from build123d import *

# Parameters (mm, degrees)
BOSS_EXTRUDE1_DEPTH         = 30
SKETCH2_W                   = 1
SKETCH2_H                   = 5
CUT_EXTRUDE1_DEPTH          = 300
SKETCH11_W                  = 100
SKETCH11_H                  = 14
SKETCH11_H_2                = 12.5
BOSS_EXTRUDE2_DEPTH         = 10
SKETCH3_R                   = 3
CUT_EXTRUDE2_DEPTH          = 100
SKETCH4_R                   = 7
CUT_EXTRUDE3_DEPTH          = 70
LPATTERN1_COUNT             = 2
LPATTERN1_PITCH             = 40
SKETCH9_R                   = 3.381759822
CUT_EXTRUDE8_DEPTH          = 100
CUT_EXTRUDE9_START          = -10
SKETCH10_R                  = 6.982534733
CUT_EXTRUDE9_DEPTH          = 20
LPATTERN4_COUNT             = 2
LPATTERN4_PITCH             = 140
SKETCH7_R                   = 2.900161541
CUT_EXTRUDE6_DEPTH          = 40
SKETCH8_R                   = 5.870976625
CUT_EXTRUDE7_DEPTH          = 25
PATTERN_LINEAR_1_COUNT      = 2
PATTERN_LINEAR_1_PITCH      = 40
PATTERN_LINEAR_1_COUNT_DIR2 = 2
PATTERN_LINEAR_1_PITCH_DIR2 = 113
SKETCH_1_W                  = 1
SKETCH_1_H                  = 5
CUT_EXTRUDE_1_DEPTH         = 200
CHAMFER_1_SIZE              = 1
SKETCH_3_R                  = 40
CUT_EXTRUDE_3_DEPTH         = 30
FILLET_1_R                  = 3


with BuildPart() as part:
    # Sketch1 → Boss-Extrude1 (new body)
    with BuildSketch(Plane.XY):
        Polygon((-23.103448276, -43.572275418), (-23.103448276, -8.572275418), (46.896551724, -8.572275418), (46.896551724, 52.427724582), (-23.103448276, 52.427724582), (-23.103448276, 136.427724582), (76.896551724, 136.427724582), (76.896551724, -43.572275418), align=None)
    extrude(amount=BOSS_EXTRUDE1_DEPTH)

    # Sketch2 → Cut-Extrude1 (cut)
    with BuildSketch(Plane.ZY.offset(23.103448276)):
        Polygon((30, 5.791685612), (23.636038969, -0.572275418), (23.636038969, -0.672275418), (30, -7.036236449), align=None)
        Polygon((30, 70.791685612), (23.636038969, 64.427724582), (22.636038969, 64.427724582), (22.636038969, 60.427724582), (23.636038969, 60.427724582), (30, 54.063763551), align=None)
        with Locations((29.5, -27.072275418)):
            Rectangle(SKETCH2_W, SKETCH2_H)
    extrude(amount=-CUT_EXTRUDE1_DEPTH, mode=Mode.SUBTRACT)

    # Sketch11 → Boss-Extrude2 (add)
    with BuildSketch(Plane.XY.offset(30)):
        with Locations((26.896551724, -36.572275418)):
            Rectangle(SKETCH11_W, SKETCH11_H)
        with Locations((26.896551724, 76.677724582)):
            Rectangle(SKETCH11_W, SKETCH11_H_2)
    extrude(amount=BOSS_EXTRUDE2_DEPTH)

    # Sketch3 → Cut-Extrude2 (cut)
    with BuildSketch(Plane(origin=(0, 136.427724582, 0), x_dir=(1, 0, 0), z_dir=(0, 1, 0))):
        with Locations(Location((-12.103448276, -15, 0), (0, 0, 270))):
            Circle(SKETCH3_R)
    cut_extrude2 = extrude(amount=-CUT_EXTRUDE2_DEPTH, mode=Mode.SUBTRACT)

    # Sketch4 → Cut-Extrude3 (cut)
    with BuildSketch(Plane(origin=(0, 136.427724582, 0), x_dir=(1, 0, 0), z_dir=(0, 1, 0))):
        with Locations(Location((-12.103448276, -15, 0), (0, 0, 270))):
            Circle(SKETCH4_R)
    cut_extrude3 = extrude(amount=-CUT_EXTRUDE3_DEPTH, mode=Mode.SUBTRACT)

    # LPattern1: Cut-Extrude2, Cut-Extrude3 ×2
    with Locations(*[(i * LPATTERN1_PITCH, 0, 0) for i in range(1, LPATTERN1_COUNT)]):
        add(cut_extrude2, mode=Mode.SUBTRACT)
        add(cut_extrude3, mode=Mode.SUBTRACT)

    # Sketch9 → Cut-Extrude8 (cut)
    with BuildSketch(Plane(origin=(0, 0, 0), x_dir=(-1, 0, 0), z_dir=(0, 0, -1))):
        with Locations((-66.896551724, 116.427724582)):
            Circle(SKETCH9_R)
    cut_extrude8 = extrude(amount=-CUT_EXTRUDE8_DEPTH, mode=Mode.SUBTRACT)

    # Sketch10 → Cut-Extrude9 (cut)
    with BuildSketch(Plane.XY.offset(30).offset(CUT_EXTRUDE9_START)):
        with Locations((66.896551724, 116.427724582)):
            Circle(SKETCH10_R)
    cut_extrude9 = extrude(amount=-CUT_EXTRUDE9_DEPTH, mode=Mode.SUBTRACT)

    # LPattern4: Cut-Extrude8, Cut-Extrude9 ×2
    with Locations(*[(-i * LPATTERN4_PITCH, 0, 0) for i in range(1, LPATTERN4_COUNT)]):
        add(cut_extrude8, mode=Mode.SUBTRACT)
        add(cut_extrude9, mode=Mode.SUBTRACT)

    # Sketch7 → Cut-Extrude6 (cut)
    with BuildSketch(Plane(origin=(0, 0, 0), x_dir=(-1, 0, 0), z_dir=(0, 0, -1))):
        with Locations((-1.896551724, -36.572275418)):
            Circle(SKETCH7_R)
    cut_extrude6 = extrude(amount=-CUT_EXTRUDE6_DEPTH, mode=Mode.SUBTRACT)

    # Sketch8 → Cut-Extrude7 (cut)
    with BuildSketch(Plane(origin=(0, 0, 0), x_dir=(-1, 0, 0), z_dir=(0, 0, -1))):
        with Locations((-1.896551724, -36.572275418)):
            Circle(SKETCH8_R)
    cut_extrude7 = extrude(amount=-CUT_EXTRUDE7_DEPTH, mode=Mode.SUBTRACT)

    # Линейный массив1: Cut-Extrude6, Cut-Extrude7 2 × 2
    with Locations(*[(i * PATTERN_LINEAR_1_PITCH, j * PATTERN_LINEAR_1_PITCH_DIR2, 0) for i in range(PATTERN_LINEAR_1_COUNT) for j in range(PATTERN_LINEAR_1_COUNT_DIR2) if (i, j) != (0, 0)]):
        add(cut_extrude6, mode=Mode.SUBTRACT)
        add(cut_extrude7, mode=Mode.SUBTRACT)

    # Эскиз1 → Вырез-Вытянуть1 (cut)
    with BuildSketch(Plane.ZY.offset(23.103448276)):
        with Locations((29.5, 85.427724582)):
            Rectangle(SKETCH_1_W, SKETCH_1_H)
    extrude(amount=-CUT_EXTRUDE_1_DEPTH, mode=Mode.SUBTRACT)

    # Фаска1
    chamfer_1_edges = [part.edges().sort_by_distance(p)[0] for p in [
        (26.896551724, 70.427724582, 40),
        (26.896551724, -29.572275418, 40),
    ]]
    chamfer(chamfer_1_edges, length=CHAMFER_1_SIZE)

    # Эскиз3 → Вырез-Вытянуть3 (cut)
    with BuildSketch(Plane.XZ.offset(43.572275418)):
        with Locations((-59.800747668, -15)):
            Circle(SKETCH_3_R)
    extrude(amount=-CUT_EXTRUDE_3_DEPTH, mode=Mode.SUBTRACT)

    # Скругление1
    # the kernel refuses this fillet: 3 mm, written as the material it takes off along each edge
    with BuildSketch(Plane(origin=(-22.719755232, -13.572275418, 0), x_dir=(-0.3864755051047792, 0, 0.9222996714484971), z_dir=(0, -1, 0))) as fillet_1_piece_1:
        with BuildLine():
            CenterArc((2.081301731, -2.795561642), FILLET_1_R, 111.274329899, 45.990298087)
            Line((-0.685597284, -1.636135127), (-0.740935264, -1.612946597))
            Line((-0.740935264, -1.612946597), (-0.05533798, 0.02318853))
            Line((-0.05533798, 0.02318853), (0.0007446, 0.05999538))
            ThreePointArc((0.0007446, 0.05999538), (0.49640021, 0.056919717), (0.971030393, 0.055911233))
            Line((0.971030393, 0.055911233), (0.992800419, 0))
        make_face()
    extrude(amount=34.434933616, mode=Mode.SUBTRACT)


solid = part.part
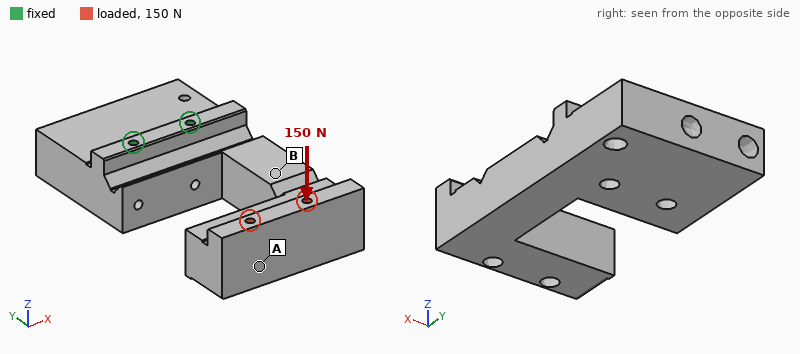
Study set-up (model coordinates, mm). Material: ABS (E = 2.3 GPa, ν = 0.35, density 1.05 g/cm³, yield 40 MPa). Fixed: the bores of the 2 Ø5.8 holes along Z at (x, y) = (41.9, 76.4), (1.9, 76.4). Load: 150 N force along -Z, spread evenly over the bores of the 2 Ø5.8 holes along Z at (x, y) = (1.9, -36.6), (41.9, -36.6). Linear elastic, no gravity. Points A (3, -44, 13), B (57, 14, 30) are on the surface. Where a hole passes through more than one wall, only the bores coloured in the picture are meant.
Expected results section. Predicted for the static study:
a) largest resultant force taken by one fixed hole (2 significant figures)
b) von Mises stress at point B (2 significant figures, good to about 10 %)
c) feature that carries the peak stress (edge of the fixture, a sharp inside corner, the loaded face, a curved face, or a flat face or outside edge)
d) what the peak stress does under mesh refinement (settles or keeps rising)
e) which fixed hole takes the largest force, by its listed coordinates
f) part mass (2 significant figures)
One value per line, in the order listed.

96 N
2.3 MPa
edge of the fixture
keeps rising
(41.9, 76.4)
410 g
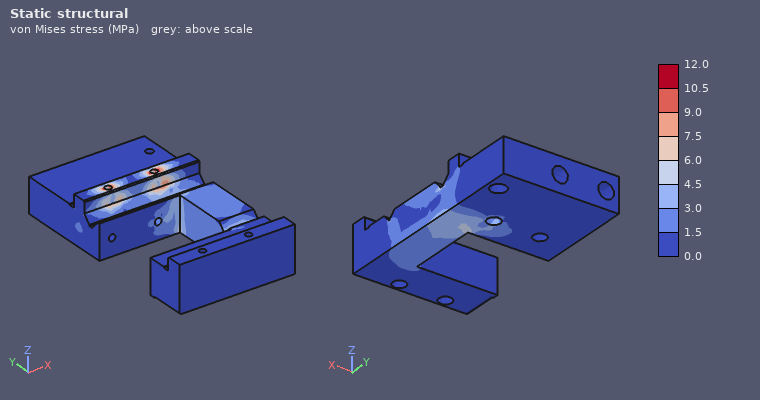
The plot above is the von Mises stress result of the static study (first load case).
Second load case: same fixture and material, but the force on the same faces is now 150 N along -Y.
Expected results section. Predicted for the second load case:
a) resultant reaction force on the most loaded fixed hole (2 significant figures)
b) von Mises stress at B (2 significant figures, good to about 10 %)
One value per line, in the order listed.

79 N
0.94 MPa
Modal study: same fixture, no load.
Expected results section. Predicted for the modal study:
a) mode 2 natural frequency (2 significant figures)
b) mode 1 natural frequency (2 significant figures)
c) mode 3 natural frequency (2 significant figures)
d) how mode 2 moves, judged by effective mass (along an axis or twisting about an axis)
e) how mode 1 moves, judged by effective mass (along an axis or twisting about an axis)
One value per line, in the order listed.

220 Hz
130 Hz
400 Hz
along X
along Z
